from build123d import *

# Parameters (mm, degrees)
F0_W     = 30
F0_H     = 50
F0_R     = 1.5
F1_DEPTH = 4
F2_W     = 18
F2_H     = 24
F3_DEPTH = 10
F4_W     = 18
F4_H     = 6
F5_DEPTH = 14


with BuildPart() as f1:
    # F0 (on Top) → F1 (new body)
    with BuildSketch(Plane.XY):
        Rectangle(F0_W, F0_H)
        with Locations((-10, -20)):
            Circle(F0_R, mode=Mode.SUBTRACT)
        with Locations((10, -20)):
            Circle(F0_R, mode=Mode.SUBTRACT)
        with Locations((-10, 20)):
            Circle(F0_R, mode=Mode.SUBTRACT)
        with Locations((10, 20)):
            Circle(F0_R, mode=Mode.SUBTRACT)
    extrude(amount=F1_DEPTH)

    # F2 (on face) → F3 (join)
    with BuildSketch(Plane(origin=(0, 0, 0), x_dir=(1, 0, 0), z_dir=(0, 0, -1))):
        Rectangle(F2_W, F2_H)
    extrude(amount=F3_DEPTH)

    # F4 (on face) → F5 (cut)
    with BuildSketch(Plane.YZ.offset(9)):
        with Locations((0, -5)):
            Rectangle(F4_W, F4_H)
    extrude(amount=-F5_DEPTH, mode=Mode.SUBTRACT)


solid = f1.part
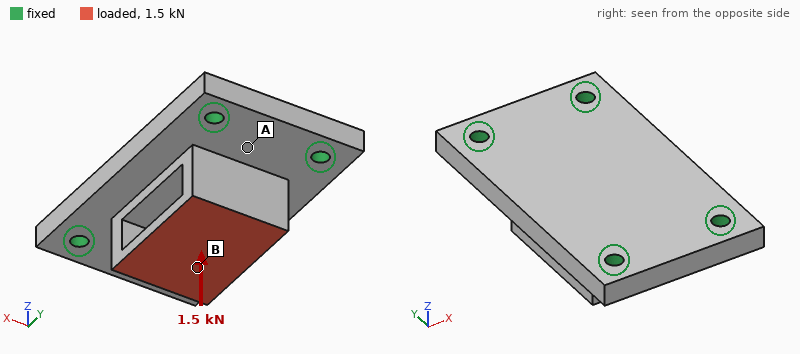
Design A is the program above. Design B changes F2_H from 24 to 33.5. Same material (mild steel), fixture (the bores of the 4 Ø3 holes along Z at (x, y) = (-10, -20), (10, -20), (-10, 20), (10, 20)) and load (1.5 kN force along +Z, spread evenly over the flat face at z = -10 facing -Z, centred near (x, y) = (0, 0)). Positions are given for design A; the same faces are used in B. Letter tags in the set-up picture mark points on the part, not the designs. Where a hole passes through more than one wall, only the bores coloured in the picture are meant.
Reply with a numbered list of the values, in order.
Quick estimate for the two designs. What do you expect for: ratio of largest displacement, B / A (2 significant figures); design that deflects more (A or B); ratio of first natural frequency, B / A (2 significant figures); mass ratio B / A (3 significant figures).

1. 0.60
2. A
3. 1.3
4. 1.20
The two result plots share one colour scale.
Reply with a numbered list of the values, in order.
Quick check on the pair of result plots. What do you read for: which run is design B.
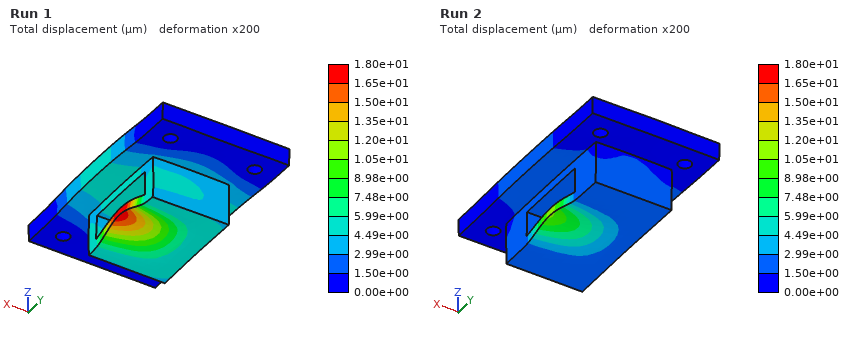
1. Run 2
